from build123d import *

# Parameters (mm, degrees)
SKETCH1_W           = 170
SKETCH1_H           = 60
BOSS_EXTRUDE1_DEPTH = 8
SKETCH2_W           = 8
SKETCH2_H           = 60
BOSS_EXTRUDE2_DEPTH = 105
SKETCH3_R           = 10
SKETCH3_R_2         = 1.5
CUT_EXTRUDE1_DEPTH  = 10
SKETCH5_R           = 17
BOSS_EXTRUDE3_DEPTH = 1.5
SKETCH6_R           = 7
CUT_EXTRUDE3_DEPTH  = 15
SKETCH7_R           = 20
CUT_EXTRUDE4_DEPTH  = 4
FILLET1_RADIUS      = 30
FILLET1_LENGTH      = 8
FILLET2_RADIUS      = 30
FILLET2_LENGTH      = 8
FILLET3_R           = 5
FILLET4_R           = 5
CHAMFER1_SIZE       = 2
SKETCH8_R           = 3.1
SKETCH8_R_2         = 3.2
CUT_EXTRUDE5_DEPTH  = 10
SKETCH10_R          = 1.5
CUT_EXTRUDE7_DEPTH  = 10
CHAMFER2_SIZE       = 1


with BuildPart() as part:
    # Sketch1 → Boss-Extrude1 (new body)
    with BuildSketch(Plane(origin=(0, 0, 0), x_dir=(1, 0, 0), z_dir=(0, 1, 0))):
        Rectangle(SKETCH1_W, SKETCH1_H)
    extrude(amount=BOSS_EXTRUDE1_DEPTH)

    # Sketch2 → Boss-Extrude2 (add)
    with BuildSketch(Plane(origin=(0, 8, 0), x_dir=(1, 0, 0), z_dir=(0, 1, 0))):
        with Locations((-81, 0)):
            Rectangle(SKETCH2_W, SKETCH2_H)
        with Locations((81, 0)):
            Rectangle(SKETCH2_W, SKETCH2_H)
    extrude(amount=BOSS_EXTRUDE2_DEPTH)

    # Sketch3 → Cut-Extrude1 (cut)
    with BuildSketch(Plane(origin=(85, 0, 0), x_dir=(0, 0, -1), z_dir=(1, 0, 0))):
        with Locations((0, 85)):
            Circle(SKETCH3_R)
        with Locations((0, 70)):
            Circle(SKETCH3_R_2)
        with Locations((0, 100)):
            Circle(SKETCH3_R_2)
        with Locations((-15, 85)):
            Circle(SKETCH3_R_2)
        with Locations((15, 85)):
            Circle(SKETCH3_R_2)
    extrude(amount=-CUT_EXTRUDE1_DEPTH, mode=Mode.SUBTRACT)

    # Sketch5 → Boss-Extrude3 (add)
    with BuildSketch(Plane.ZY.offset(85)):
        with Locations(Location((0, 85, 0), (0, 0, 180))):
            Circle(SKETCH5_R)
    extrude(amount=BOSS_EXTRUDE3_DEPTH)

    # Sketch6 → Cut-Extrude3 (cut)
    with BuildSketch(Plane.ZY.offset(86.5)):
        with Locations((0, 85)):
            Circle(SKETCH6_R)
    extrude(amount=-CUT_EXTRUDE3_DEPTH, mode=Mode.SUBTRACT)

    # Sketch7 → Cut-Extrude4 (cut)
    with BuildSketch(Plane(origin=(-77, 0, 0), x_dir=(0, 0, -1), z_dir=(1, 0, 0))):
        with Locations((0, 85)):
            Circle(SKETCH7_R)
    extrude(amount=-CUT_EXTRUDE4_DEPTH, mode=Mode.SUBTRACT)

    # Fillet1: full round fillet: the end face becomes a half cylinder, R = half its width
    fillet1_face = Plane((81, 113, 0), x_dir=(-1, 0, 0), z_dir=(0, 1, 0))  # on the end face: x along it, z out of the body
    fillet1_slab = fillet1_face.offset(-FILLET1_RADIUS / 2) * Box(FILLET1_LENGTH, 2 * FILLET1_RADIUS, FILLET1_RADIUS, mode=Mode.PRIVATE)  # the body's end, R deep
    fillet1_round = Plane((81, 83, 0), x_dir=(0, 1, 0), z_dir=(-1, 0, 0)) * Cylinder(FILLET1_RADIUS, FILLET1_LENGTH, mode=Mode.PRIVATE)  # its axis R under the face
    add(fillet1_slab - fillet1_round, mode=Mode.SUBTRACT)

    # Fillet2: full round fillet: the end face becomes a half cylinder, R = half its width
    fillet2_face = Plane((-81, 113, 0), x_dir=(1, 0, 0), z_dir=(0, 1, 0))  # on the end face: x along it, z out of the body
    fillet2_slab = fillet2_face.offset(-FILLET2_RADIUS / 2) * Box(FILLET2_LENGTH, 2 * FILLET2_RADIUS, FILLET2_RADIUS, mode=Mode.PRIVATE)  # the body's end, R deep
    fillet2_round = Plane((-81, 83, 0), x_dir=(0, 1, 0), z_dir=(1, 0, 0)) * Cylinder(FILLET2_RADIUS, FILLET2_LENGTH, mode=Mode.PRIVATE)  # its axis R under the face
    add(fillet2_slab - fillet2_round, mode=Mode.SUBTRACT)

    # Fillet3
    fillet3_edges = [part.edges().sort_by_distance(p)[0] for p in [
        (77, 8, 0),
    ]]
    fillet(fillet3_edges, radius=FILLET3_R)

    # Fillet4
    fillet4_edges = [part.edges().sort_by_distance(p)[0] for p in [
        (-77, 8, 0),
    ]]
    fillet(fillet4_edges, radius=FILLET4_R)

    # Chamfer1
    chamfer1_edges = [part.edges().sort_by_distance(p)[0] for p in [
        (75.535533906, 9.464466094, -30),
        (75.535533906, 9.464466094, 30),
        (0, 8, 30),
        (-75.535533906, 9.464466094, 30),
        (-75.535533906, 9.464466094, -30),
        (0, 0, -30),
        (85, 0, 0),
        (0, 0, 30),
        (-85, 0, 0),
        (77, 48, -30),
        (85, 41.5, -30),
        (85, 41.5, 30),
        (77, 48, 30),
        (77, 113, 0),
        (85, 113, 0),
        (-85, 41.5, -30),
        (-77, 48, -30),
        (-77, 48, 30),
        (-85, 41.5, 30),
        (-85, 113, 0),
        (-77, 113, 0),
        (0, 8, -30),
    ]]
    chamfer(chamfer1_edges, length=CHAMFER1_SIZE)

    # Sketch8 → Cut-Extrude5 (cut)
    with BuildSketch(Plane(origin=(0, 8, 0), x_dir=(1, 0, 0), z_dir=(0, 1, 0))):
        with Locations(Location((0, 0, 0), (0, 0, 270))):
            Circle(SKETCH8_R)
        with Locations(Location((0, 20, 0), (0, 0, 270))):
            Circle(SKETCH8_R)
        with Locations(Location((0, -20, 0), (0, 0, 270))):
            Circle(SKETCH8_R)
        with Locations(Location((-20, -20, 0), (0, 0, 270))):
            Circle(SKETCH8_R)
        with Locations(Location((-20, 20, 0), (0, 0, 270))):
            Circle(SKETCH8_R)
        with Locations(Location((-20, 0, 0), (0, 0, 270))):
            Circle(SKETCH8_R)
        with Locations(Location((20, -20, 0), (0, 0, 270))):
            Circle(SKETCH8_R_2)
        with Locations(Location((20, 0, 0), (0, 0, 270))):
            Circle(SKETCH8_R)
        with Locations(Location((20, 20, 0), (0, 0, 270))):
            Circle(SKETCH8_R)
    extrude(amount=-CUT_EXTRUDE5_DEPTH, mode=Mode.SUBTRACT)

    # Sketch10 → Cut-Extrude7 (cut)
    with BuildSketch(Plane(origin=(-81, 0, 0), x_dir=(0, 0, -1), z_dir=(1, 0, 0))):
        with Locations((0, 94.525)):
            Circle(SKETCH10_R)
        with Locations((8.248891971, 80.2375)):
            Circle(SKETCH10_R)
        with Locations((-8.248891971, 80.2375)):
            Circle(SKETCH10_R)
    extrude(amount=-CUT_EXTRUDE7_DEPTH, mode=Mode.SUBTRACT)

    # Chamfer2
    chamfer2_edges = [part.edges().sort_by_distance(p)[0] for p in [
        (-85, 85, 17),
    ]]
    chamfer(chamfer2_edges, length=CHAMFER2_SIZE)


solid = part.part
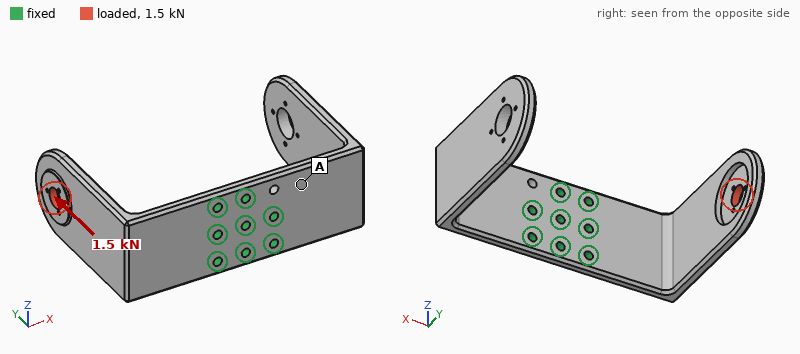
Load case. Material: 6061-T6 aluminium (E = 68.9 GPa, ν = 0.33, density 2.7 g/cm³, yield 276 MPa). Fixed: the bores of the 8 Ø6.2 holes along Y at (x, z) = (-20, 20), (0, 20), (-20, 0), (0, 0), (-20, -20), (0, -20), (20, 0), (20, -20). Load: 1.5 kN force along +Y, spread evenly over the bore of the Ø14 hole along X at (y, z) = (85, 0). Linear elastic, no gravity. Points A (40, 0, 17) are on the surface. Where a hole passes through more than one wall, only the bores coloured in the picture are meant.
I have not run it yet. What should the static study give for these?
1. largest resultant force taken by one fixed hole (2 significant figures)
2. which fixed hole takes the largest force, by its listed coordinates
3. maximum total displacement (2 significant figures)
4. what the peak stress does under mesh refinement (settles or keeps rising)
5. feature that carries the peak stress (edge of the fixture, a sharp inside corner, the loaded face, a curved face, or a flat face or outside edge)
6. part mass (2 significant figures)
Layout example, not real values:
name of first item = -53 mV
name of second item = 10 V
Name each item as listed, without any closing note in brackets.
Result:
largest resultant force taken by one fixed hole = 1.3 kN
which fixed hole takes the largest force, by its listed coordinates = (-20, 0)
maximum total displacement = 2.0 mm
what the peak stress does under mesh refinement = keeps rising
feature that carries the peak stress = edge of the fixture
part mass = 440 g
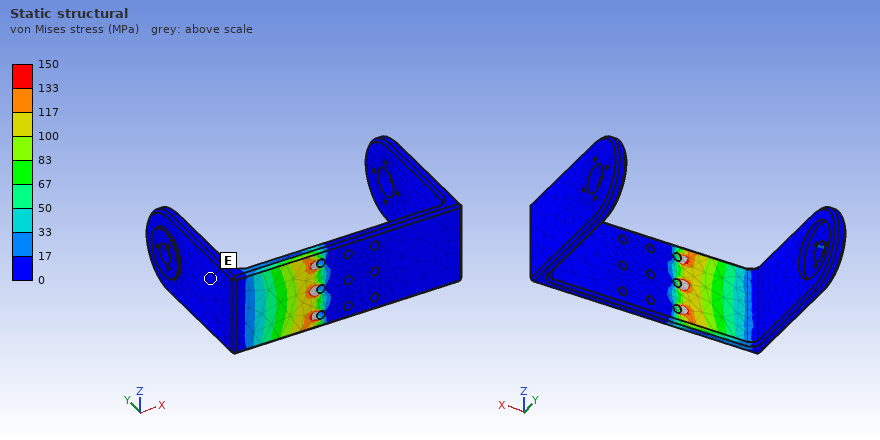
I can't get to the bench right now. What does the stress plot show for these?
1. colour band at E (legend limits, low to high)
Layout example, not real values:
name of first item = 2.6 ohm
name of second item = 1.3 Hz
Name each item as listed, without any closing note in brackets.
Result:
colour band at E = 0 to 17 MPa
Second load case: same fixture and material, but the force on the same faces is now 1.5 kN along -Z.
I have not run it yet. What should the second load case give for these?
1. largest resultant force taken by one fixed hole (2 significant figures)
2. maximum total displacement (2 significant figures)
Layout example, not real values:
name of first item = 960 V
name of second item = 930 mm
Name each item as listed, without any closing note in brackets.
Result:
largest resultant force taken by one fixed hole = 3.5 kN
maximum total displacement = 2.1 mm
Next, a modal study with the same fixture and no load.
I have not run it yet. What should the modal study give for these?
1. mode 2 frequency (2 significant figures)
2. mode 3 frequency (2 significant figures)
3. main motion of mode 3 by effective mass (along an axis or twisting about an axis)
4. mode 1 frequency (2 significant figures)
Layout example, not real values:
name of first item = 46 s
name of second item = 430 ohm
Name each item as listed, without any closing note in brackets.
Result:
mode 2 frequency = 360 Hz
mode 3 frequency = 550 Hz
main motion of mode 3 by effective mass = along Z
mode 1 frequency = 340 Hz
